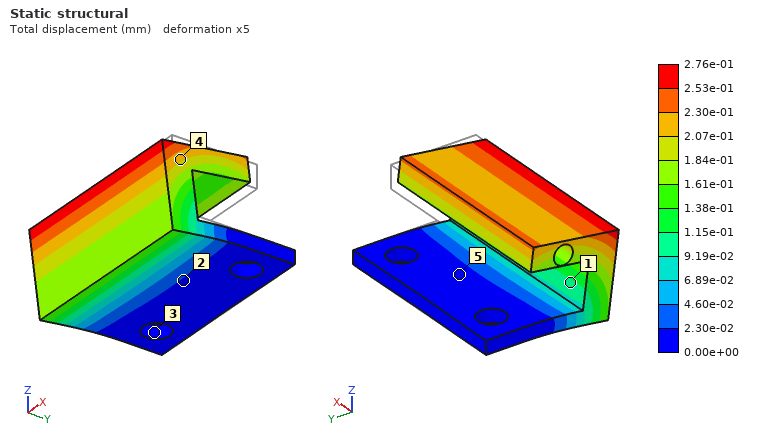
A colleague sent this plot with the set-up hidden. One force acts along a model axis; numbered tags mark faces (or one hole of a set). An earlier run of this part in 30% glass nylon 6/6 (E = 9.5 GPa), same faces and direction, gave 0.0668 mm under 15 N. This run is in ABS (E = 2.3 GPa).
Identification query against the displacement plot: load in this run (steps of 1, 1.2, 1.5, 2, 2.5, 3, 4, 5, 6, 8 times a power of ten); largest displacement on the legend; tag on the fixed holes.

15 N
2.76e-01 mm
3
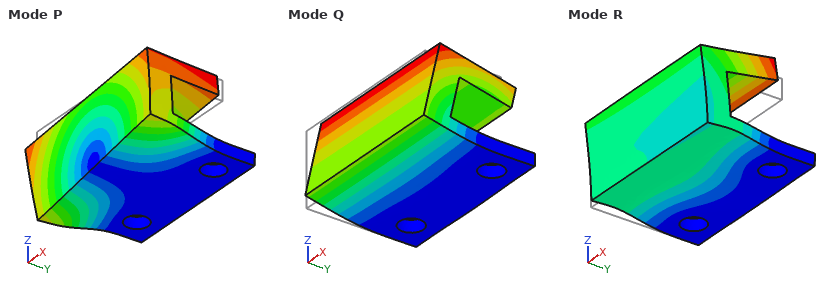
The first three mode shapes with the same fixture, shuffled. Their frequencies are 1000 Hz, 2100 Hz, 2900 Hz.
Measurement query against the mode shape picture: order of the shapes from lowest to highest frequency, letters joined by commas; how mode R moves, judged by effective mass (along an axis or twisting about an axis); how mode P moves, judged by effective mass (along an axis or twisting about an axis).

Q, P, R
along Z
along X
